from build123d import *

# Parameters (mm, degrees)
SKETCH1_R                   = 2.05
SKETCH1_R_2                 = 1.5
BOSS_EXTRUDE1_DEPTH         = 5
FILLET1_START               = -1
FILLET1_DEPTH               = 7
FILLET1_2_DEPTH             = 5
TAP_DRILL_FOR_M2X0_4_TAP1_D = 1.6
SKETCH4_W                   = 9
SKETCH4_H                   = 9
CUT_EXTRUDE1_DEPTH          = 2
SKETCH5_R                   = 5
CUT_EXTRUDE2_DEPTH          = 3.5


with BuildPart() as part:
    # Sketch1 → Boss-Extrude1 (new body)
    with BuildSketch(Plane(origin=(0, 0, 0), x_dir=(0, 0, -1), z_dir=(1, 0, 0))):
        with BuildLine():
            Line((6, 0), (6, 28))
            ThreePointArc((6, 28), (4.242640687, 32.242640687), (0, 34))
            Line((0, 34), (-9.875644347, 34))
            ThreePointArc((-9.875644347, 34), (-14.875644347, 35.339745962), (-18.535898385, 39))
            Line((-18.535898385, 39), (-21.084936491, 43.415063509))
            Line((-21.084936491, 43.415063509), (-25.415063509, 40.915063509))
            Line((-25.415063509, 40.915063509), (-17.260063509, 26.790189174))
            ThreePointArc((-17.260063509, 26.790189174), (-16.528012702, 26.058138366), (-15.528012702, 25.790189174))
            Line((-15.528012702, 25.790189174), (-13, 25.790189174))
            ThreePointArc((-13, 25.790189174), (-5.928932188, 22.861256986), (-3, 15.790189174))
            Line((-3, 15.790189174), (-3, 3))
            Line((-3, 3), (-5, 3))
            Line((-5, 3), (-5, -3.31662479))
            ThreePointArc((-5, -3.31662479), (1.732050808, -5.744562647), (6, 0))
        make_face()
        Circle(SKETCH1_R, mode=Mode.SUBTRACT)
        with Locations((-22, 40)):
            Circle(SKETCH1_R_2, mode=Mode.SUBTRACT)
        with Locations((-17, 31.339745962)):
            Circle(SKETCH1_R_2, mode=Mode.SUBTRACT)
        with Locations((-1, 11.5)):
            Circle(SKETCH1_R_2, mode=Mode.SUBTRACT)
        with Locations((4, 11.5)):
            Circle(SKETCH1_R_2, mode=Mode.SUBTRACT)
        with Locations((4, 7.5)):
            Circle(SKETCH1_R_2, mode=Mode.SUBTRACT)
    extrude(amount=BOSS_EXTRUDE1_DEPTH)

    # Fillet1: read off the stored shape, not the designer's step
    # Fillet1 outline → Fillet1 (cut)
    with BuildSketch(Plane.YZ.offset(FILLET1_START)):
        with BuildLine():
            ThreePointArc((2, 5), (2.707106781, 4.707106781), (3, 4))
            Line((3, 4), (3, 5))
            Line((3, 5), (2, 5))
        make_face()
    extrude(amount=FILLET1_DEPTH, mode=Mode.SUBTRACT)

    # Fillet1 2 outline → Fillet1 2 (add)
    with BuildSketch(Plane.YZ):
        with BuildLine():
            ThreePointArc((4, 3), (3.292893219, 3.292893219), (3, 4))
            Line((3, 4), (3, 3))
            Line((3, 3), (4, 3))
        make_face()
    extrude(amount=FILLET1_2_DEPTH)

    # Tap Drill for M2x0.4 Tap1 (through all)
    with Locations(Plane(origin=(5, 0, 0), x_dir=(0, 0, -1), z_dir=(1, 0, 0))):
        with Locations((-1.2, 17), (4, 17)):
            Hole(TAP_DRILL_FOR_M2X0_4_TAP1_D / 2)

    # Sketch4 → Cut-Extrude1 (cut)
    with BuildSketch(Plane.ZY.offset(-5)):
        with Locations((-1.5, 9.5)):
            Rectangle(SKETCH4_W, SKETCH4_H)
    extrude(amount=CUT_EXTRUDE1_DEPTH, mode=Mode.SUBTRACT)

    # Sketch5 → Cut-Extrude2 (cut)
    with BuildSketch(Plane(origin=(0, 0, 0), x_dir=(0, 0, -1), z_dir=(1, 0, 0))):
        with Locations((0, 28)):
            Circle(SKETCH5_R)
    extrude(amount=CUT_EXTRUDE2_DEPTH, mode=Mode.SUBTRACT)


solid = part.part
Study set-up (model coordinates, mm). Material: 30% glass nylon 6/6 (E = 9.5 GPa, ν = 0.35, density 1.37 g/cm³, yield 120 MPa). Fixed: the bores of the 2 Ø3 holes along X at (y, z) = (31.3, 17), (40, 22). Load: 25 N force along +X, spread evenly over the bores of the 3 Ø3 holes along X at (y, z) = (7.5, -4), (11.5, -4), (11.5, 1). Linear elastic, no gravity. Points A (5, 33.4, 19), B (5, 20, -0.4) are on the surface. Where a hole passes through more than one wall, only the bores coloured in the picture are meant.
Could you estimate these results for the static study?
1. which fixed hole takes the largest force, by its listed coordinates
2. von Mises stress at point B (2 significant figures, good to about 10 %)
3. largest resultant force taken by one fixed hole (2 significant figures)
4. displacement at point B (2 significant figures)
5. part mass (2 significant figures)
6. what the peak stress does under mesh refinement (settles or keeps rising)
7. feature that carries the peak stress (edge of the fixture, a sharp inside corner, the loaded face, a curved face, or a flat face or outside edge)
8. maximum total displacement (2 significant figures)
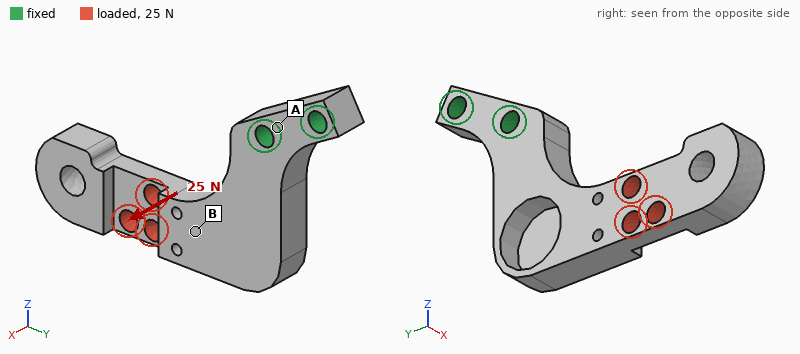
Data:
(31.3, 17)
7.6 MPa
34 N
0.17 mm
3.0 g
keeps rising
edge of the fixture
0.63 mm
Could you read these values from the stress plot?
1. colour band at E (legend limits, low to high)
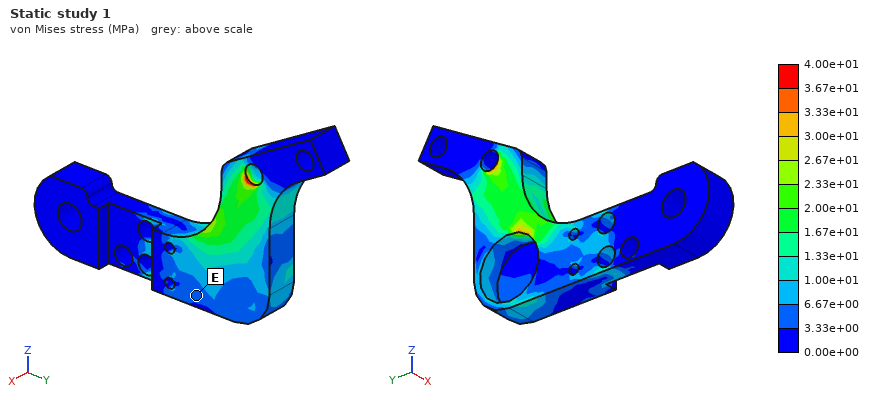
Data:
3.33e+00 to 6.67e+00 MPa
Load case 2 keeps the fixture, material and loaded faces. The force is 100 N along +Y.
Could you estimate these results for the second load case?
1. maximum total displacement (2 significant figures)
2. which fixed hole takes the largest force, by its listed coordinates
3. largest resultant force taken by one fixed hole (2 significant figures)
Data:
0.53 mm
(31.3, 17)
120 N
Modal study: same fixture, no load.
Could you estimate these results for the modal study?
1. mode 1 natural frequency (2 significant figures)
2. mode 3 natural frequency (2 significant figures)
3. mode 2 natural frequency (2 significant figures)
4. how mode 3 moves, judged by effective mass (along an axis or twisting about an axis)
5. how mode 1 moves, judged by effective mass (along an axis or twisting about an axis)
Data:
900 Hz
2900 Hz
1600 Hz
along X
along X
